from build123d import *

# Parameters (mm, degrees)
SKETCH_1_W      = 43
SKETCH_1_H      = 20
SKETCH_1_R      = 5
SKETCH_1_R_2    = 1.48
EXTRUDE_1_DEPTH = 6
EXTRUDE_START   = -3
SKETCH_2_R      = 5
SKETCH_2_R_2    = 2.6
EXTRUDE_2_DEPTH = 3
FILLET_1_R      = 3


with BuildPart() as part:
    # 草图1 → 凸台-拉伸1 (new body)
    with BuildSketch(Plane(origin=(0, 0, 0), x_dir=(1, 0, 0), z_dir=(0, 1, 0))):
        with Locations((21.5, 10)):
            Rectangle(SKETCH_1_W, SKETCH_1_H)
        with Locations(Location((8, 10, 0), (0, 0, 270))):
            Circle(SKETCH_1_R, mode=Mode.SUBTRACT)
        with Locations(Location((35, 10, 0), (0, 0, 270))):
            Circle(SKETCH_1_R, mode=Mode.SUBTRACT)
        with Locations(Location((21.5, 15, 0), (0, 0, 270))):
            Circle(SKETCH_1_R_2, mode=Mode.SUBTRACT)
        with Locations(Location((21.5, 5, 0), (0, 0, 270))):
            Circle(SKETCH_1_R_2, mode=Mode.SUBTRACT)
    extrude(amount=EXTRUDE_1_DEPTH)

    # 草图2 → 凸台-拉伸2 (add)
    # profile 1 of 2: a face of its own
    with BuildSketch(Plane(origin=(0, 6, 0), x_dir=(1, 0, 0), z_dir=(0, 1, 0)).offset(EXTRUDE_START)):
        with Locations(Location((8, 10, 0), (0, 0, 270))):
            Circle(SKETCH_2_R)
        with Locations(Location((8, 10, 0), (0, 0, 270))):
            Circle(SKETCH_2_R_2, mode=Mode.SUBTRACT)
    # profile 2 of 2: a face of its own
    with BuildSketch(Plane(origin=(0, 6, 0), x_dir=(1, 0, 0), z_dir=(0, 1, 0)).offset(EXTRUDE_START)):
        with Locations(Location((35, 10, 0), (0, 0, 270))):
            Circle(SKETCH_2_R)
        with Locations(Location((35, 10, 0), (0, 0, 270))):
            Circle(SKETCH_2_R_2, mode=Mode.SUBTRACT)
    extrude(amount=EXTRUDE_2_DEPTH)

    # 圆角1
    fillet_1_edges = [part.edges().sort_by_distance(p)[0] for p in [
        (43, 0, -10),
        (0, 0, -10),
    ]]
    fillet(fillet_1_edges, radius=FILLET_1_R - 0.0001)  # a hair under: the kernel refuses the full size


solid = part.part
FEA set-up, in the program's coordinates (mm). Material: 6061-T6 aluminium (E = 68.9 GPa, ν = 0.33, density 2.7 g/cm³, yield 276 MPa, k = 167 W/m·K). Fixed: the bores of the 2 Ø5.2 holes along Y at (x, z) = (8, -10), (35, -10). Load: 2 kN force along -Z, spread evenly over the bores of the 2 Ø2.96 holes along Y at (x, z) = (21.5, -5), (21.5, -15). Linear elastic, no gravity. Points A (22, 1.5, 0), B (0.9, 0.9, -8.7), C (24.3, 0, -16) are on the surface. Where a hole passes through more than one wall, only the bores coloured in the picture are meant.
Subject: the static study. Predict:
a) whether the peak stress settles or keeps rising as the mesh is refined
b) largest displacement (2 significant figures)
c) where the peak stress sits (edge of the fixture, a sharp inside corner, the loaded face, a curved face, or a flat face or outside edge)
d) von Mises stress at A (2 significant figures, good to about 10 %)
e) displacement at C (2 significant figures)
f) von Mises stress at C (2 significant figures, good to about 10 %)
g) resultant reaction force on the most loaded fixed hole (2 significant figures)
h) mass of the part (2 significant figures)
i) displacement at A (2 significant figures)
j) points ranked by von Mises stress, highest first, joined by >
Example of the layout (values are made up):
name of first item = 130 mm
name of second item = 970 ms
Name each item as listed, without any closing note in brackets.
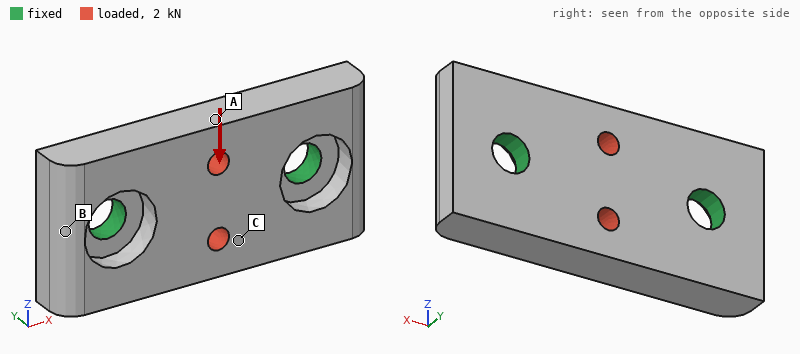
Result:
whether the peak stress settles or keeps rising as the mesh is refined = keeps rising
largest displacement = 13 µm
where the peak stress sits = edge of the fixture
von Mises stress at A = 36 MPa
displacement at C = 11 µm
von Mises stress at C = 18 MPa
resultant reaction force on the most loaded fixed hole = 1.0 kN
mass of the part = 12 g
displacement at A = 12 µm
points ranked by von Mises stress, highest first, joined by > = A > C > B
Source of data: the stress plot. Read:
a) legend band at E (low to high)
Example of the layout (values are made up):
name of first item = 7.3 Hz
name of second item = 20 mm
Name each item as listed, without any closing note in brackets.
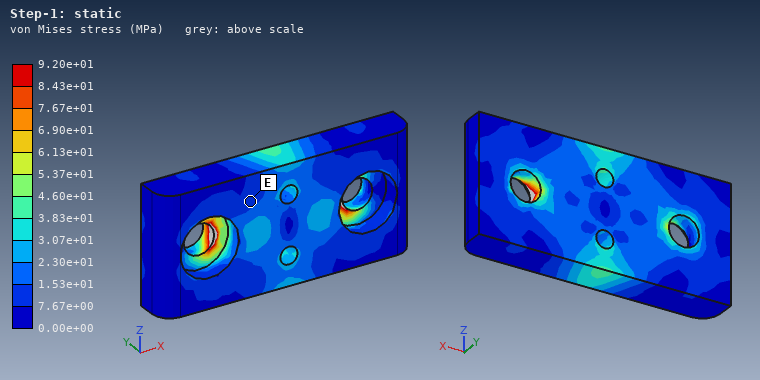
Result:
legend band at E = 7.67e+00 to 1.53e+01 MPa
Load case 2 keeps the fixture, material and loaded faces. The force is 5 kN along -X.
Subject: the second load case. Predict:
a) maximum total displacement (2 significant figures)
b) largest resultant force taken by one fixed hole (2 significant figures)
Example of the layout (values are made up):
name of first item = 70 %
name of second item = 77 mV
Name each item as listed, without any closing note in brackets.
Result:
maximum total displacement = 8.4 µm
largest resultant force taken by one fixed hole = 2.5 kN
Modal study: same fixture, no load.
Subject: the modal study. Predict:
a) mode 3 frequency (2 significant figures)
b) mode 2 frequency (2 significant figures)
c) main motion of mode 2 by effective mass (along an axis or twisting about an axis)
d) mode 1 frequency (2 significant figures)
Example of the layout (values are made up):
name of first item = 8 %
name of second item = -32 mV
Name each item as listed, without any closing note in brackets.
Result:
mode 3 frequency = 27 kHz
mode 2 frequency = 24 kHz
main motion of mode 2 by effective mass = along Y
mode 1 frequency = 18 kHz
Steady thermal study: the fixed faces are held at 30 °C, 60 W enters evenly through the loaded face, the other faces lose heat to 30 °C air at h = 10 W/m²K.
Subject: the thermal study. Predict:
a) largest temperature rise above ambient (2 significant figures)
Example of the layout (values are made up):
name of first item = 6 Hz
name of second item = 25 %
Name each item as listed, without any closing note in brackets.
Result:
largest temperature rise above ambient = 27 K
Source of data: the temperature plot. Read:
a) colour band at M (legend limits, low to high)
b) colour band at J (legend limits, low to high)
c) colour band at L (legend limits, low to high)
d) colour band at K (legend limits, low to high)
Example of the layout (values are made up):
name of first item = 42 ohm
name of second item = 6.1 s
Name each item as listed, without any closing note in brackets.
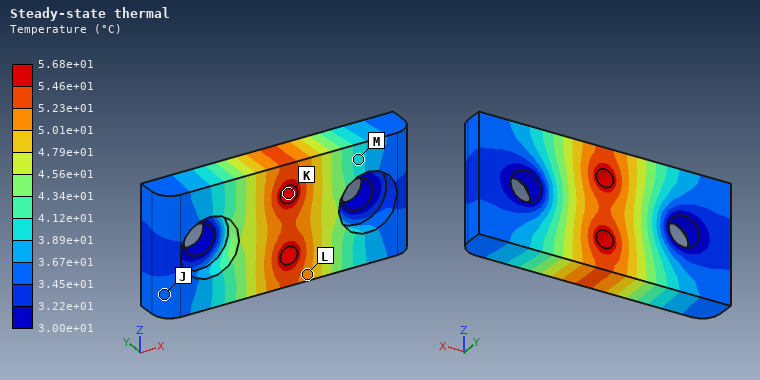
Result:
colour band at M = 3.89e+01 to 4.12e+01 °C
colour band at J = 3.45e+01 to 3.67e+01 °C
colour band at L = 5.01e+01 to 5.23e+01 °C
colour band at K = 5.46e+01 to 5.68e+01 °C
